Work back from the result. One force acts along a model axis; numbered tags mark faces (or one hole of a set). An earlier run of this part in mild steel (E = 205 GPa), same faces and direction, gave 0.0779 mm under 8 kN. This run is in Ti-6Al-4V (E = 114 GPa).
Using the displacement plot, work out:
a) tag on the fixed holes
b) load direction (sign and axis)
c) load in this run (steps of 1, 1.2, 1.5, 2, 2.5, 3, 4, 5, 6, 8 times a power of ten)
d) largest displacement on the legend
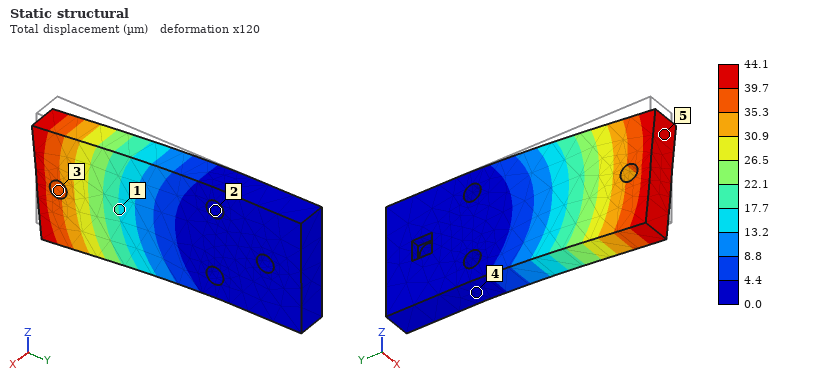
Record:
2
-Z
2.5 kN
44.1 µm
